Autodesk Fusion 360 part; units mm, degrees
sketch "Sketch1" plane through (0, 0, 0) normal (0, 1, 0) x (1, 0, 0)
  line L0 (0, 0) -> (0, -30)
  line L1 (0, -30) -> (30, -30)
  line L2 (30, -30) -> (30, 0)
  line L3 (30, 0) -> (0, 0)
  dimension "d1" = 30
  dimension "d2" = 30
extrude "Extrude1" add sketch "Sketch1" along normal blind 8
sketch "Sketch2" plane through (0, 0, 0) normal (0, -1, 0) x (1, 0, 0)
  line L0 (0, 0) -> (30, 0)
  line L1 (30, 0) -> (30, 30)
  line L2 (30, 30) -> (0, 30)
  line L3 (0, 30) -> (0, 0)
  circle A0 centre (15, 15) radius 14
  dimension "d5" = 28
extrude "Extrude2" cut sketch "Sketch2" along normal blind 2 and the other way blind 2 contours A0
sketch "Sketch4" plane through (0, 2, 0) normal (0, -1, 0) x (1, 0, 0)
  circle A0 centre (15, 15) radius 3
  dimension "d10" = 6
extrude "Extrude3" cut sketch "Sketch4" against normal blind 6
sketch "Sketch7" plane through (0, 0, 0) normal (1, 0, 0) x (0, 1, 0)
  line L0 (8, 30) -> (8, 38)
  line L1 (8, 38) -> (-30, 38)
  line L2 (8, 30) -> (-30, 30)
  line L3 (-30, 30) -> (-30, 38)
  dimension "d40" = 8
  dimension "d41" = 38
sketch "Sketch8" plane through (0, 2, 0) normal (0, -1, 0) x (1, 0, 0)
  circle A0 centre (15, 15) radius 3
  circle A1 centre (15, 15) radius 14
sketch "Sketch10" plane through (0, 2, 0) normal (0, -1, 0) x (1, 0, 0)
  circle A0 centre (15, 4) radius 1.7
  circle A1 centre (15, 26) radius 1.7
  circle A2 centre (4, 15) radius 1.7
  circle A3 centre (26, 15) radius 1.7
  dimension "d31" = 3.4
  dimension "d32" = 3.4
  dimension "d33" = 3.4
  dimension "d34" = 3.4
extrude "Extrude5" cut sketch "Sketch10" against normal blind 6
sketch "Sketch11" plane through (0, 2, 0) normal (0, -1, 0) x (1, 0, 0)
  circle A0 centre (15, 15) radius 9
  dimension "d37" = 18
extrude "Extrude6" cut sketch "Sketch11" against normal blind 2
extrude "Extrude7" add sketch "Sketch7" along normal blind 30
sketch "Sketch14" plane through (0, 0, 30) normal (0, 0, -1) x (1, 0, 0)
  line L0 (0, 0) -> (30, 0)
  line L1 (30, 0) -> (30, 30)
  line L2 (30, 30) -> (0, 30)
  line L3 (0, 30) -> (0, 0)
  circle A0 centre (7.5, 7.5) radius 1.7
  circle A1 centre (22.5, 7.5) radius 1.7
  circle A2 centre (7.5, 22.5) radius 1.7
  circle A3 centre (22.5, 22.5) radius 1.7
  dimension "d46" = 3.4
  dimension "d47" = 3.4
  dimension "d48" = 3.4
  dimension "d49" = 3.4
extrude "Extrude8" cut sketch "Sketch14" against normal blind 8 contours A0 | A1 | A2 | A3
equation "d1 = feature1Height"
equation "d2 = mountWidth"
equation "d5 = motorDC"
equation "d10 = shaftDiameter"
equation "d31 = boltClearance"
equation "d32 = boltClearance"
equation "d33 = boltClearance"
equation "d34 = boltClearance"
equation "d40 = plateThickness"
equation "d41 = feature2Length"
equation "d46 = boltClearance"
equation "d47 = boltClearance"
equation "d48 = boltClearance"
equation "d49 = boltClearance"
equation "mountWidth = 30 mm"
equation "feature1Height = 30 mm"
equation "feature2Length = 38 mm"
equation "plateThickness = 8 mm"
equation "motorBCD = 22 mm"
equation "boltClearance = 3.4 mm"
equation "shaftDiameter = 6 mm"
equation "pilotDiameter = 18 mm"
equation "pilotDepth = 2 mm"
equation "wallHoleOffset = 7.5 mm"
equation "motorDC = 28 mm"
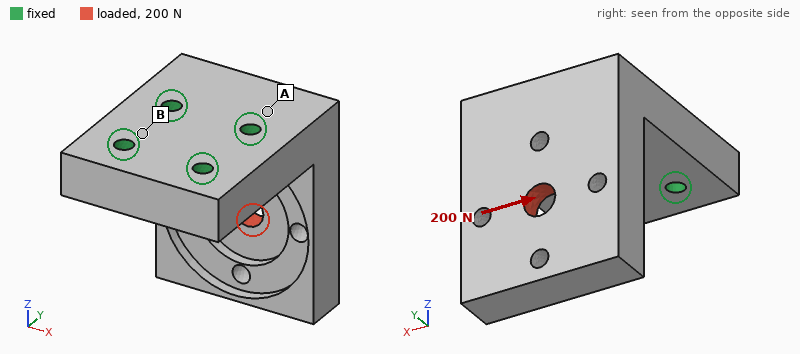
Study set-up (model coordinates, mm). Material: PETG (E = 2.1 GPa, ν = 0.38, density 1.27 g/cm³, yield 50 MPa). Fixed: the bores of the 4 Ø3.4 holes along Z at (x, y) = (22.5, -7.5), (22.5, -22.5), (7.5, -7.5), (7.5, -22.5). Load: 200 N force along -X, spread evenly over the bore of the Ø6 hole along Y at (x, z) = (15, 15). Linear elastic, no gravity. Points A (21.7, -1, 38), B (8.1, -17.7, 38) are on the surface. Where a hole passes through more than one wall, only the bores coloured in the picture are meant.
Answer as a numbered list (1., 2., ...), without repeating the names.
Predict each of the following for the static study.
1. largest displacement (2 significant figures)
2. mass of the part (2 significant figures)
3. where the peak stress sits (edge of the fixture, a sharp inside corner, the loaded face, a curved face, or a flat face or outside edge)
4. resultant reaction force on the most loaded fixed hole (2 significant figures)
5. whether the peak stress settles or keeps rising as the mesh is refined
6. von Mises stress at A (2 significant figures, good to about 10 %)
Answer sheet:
1. 0.33 mm
2. 18 g
3. edge of the fixture
4. 240 N
5. keeps rising
6. 3.2 MPa
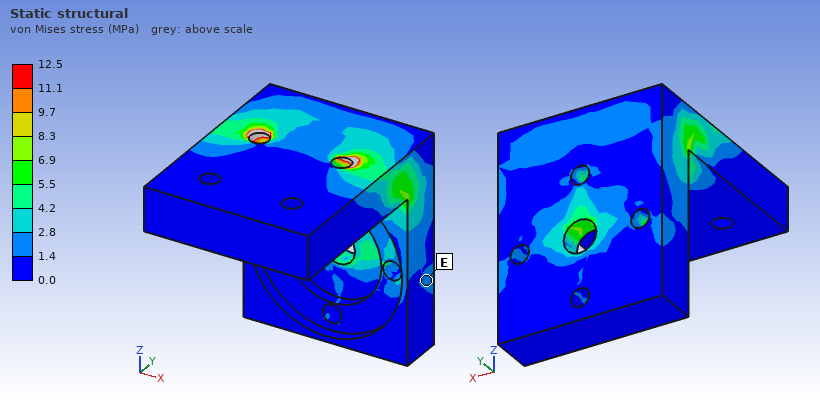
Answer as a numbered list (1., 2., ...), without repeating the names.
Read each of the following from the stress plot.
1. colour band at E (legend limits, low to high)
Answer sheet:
1. 1.4 to 2.8 MPa
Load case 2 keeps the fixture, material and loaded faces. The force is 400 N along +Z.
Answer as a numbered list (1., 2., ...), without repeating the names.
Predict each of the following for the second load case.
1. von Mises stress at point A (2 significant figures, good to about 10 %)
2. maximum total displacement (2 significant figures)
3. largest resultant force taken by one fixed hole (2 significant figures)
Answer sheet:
1. 8.7 MPa
2. 0.64 mm
3. 240 N
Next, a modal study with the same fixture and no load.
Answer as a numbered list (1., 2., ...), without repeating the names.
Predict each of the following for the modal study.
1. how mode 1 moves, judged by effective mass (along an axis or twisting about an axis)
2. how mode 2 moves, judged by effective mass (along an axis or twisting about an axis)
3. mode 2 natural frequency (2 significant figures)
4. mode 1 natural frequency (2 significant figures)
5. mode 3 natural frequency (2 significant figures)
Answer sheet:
1. along Y
2. along X
3. 1600 Hz
4. 960 Hz
5. 2500 Hz
